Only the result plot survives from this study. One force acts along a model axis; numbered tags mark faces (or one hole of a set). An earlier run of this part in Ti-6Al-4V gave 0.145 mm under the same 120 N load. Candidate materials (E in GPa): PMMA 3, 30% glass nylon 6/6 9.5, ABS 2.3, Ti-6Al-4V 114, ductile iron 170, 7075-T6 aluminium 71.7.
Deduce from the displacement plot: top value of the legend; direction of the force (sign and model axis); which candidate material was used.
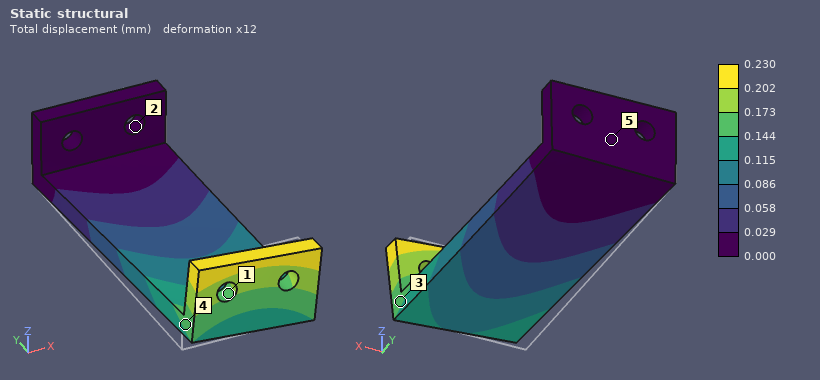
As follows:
0.230 mm
+X
7075-T6 aluminium
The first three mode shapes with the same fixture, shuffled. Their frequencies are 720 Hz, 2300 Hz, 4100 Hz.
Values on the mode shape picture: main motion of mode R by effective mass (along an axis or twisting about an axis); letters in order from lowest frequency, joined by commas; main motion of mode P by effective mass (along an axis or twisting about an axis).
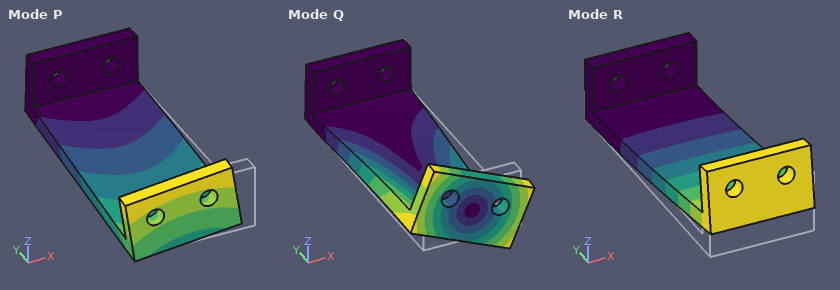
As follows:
along Z
R, P, Q
along X
